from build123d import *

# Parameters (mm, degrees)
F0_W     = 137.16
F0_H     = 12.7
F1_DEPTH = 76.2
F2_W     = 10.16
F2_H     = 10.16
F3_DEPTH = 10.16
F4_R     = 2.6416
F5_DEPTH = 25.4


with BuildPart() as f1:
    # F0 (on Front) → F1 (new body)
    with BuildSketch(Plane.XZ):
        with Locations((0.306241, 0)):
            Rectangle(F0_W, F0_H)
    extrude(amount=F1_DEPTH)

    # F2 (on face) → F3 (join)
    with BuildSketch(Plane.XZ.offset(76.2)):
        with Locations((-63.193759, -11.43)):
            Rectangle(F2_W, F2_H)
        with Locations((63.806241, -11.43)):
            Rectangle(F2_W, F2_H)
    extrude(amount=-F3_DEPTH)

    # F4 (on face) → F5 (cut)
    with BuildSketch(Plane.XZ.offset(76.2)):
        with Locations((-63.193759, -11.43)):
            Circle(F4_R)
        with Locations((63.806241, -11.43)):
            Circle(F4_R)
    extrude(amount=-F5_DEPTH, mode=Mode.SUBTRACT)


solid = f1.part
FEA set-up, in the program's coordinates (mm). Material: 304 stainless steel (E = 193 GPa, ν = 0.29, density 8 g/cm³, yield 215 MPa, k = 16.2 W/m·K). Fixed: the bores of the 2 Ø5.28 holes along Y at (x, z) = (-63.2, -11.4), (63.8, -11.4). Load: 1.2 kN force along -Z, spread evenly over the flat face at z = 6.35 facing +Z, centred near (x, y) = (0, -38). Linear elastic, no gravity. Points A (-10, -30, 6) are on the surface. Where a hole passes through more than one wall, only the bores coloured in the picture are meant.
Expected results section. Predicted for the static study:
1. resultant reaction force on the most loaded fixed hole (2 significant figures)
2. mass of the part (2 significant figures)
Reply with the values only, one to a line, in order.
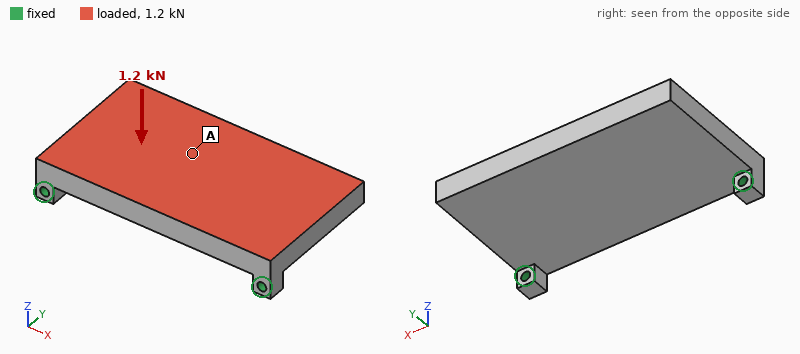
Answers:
740 N
1.1 kg
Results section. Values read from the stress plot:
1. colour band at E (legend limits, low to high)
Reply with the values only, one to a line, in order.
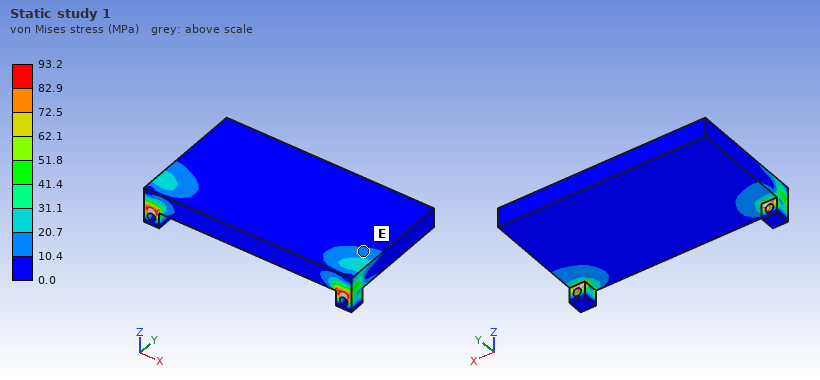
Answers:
10.4 to 20.7 MPa
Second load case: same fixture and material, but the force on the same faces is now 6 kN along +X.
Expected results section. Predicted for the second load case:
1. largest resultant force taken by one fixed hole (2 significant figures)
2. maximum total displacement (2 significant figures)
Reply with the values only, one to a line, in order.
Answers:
3.4 kN
12 µm
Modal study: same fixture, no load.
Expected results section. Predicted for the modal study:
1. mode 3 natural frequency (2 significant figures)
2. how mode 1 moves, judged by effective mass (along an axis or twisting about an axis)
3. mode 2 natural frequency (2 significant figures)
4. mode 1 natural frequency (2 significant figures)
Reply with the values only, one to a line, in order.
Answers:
3100 Hz
along Z
2200 Hz
670 Hz
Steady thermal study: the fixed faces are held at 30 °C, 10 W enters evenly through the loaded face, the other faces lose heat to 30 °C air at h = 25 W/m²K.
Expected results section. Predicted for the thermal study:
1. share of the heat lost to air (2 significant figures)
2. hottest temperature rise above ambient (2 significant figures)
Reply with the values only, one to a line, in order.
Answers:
61 %
18 K
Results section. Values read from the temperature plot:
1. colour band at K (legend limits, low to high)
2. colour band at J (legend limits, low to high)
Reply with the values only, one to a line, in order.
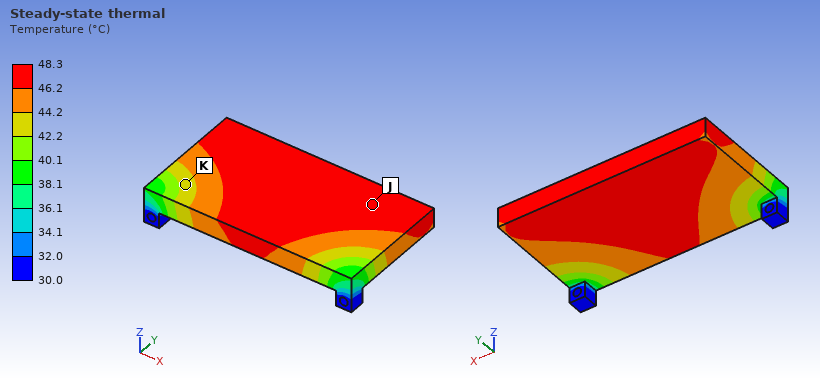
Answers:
42.2 to 44.2 °C
46.2 to 48.3 °C
